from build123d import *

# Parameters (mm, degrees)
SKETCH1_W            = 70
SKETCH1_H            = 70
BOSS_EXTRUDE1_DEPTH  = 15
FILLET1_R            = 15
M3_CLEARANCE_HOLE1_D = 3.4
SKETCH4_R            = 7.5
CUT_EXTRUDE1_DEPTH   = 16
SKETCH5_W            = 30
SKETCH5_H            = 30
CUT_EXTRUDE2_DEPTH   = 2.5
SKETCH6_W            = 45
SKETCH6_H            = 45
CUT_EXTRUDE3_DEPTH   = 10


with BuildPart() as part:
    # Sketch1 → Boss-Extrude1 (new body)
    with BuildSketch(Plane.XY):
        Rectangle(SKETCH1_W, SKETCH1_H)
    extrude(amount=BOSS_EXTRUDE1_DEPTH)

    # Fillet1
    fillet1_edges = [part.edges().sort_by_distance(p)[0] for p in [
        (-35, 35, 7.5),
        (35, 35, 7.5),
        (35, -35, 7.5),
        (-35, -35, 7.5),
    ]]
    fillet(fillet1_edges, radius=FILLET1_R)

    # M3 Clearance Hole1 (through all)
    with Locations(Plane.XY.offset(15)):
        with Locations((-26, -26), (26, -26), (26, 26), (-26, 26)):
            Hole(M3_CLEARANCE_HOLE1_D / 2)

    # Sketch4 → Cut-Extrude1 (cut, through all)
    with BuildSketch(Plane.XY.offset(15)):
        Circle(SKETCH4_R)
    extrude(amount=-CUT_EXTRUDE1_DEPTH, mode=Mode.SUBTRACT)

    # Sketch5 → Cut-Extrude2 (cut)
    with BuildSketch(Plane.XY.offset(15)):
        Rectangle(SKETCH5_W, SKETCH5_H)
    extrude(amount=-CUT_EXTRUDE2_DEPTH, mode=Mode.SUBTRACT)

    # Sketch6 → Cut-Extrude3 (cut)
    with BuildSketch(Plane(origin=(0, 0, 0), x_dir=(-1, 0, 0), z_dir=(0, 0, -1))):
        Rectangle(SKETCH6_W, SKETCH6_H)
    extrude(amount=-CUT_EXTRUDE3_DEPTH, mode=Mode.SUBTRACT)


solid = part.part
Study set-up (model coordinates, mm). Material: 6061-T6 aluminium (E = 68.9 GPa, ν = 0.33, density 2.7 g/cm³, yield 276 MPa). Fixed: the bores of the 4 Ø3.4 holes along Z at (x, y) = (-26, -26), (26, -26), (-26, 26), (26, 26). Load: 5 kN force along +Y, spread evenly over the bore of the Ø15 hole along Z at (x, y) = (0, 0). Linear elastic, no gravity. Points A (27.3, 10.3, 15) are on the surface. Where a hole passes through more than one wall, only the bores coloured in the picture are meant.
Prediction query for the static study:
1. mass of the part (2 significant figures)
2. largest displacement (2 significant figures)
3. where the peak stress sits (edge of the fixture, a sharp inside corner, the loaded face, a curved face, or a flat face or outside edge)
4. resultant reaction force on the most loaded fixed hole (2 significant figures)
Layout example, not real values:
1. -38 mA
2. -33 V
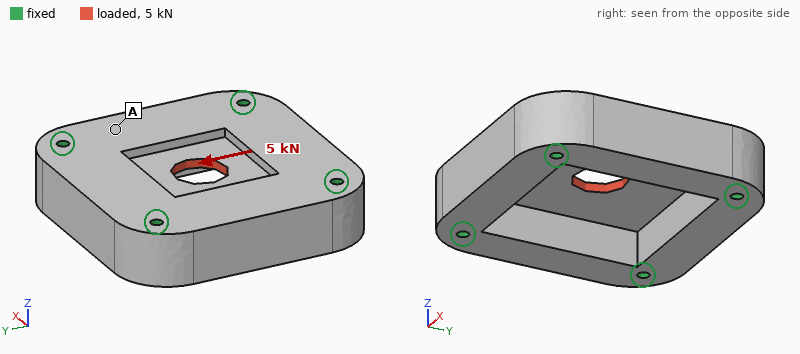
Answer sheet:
1. 130 g
2. 12 µm
3. the loaded face
4. 1.3 kN
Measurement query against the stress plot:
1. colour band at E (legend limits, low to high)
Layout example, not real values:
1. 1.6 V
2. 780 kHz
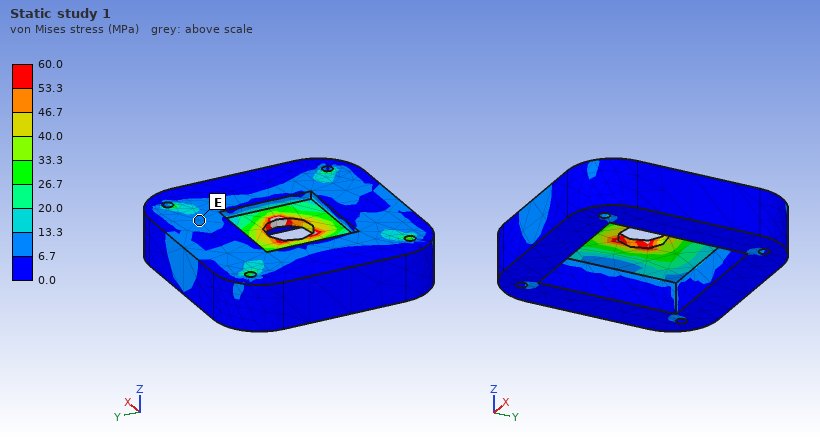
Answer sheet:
1. 6.7 to 13.3 MPa
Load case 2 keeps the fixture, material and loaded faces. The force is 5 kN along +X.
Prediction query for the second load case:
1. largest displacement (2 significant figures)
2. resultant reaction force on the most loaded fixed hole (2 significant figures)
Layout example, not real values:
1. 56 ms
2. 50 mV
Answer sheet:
1. 12 µm
2. 1.3 kN
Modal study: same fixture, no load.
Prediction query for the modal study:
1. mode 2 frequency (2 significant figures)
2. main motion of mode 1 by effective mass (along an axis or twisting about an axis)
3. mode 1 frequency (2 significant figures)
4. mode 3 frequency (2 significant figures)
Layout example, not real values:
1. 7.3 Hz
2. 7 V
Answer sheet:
1. 17 kHz
2. along Z
3. 13 kHz
4. 17 kHz
